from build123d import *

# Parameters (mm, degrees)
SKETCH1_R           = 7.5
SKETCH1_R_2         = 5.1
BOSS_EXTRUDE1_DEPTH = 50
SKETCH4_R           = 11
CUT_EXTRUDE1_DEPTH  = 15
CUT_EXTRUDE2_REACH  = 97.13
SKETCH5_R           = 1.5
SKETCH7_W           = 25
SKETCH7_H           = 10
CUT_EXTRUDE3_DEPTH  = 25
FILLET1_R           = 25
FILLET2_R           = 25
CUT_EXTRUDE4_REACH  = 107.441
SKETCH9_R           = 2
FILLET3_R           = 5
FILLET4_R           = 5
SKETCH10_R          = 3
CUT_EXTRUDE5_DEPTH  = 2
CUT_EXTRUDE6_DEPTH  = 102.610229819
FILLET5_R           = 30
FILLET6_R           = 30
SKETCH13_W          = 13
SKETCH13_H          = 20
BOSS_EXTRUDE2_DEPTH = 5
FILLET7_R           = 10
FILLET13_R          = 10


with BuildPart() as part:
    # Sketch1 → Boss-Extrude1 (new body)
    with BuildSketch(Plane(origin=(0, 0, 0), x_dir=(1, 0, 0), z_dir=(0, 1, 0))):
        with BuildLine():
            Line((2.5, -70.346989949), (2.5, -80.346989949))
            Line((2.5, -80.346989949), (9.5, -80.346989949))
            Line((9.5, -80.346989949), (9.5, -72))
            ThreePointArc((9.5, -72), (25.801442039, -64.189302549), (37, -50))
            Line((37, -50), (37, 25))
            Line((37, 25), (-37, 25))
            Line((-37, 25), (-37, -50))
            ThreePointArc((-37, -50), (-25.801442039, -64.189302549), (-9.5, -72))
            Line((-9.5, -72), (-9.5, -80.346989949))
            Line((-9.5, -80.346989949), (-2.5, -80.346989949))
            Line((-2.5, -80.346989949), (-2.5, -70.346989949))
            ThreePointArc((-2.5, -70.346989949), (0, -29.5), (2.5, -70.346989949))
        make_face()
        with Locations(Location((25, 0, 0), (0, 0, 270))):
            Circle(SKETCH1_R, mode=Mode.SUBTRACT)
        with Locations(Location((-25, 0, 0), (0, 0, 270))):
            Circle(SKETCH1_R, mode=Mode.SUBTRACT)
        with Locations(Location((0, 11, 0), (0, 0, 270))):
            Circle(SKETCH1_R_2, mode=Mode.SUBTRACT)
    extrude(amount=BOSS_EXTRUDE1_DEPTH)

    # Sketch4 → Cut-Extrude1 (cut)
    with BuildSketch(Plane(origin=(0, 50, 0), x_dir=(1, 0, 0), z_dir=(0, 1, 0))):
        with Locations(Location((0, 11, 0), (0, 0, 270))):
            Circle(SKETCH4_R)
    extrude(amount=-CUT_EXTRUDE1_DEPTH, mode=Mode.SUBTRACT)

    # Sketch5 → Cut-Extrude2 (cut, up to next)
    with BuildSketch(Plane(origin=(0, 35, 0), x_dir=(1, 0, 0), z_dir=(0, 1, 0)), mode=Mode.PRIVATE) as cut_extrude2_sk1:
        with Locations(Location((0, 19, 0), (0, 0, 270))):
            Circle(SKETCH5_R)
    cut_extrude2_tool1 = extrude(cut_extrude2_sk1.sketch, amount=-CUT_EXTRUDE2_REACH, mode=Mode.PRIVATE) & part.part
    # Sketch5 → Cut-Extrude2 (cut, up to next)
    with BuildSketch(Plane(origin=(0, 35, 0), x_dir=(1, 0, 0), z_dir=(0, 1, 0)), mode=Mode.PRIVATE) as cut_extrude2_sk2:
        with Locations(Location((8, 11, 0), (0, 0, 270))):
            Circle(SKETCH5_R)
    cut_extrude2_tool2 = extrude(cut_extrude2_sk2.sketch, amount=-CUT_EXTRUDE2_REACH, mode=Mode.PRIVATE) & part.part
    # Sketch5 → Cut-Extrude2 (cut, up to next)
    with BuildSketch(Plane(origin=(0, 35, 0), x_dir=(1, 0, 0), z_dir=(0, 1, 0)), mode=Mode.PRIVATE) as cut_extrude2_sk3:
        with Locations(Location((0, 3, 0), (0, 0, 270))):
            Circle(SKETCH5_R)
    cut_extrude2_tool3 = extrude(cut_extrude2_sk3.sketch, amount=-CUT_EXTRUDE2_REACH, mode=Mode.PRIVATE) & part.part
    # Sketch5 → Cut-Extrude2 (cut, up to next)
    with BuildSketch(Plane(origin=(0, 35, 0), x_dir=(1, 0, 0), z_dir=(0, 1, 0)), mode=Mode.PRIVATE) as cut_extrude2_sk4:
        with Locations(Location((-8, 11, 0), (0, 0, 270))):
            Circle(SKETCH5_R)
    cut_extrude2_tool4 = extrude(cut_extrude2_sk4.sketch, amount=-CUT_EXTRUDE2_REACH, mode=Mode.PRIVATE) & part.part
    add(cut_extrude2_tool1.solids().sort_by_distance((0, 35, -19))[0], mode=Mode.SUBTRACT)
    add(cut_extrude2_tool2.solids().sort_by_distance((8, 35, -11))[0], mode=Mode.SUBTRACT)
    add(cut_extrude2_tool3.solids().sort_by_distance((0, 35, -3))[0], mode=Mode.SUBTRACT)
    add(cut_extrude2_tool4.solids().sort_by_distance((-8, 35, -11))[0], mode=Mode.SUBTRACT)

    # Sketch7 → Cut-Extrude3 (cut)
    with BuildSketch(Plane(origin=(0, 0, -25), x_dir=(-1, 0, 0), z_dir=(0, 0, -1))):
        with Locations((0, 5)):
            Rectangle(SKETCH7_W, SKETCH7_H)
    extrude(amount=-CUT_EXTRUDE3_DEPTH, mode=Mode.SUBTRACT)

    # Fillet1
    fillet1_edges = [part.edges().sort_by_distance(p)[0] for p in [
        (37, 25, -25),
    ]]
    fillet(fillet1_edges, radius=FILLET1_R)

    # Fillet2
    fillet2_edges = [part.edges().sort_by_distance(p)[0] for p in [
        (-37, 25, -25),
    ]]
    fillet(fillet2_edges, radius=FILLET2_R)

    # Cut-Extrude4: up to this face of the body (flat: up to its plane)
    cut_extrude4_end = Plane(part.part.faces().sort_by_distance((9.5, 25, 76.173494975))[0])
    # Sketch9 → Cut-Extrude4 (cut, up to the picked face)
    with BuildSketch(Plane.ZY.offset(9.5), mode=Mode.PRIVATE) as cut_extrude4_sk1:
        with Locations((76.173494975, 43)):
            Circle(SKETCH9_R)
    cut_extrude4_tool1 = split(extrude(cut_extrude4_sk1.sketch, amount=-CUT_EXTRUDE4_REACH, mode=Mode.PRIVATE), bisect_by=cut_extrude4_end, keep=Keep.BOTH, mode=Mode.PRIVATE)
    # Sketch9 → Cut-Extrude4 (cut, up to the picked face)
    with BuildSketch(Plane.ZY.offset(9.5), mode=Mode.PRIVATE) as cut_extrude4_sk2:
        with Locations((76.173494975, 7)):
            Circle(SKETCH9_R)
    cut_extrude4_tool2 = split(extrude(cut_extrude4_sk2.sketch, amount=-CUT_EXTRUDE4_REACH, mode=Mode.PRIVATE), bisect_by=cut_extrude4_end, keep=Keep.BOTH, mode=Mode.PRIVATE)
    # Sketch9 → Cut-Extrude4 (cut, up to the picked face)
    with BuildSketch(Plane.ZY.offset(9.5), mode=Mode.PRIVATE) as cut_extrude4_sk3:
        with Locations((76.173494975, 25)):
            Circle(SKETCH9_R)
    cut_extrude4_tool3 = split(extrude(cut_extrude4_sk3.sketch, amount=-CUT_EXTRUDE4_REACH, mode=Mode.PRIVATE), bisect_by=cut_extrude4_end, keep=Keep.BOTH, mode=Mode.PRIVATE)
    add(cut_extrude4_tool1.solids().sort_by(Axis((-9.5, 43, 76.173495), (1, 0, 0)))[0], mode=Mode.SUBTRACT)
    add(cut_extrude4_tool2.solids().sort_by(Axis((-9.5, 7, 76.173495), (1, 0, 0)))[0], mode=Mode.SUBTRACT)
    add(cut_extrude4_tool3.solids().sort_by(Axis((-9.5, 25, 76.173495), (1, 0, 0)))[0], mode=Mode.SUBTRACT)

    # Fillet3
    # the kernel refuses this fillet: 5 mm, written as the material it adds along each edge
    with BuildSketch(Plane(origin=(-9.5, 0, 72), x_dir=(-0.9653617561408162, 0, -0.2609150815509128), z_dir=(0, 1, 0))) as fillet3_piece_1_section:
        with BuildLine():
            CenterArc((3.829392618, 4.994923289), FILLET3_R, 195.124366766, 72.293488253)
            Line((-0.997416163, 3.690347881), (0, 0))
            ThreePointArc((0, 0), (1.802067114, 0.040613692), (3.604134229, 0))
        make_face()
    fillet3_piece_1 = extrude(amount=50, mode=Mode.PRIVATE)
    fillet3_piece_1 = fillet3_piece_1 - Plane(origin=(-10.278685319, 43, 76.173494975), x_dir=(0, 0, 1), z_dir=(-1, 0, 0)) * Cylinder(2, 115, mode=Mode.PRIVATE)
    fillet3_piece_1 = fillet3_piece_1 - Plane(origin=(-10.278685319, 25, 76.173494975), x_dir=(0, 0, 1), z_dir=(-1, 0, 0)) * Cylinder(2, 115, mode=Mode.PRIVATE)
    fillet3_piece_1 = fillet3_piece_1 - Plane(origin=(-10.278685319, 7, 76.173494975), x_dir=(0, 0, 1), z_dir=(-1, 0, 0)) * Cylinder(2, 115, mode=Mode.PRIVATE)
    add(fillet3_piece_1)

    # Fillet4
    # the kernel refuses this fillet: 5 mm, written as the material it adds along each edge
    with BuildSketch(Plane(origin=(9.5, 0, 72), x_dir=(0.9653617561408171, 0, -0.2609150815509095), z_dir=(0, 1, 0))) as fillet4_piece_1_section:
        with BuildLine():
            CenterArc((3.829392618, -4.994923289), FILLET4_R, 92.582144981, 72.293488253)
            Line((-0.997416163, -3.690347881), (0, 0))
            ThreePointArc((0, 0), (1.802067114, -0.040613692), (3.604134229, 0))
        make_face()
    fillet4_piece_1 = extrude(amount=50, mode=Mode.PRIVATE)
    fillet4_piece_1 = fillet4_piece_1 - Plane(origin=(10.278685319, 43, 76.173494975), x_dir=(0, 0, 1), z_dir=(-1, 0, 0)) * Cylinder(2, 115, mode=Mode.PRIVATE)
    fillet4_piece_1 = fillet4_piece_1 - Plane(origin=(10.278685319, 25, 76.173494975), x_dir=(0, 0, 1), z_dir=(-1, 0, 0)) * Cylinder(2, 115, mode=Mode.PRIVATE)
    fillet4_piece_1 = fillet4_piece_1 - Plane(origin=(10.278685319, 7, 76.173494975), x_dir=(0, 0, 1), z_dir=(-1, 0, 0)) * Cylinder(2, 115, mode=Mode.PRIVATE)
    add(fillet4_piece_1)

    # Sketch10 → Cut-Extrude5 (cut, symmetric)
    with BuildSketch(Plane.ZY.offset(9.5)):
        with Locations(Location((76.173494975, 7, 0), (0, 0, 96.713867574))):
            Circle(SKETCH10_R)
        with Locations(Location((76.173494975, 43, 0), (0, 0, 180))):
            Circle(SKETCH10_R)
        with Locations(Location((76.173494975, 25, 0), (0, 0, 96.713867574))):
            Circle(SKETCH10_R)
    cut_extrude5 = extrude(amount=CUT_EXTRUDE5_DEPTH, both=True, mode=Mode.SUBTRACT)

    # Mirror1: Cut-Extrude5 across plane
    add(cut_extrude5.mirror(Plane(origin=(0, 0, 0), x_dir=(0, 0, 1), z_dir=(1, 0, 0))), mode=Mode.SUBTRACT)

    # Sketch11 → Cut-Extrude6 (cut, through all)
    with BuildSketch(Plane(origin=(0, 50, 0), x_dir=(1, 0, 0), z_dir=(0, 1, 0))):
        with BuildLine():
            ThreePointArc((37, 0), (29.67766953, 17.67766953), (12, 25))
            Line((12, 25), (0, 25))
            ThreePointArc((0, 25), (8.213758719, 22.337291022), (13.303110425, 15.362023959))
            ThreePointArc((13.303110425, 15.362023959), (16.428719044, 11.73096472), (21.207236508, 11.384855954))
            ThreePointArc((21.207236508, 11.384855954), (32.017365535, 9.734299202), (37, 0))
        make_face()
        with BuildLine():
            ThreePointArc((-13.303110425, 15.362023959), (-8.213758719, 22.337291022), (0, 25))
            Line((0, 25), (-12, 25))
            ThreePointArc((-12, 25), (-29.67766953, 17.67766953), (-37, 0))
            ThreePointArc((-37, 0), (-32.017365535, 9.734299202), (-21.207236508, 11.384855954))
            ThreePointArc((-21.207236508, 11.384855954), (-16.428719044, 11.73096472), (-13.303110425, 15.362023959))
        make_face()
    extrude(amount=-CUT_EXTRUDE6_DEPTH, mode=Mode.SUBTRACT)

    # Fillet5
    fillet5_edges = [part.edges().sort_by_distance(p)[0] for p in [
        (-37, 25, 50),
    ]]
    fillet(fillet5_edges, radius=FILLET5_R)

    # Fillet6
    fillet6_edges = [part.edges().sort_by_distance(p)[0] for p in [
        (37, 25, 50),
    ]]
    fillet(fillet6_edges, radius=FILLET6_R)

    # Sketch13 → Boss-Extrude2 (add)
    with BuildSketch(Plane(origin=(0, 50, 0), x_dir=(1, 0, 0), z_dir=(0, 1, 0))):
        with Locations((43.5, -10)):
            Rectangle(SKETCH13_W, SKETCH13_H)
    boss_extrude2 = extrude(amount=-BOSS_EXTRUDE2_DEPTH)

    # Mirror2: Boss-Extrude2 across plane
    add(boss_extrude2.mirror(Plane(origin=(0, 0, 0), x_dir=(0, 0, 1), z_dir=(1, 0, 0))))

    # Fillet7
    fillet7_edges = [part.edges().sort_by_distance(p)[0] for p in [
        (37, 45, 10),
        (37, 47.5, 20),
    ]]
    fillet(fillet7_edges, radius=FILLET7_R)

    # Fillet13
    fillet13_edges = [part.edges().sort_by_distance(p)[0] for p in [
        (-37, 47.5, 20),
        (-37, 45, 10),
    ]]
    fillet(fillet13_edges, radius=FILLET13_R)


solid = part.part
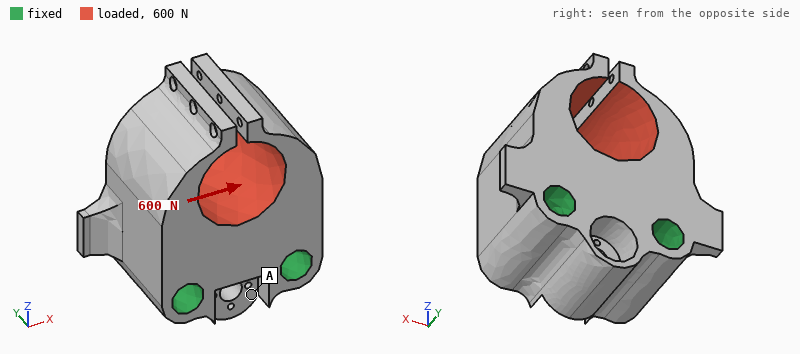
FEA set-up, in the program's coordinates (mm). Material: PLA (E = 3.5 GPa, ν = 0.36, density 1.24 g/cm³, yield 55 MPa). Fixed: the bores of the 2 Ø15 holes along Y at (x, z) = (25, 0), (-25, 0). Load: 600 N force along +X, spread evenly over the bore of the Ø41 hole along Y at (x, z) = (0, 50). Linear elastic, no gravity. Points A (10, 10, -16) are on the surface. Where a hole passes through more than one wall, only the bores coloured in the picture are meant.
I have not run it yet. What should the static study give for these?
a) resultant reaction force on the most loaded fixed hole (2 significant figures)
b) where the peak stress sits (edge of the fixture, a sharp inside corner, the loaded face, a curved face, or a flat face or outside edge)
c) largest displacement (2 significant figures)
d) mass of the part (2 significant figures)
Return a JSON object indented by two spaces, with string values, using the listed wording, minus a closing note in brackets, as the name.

{
  "resultant reaction force on the most loaded fixed hole": "540 N",
  "where the peak stress sits": "the loaded face",
  "largest displacement": "85 µm",
  "mass of the part": "260 g"
}
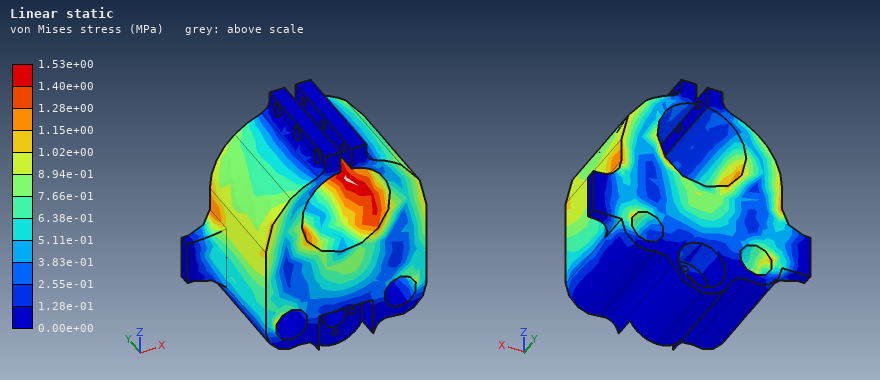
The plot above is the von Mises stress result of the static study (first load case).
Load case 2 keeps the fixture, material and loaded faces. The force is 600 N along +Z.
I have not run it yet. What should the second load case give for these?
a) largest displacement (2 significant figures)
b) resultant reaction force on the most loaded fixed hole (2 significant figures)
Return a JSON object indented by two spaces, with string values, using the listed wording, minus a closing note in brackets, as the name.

{
  "largest displacement": "0.10 mm",
  "resultant reaction force on the most loaded fixed hole": "330 N"
}
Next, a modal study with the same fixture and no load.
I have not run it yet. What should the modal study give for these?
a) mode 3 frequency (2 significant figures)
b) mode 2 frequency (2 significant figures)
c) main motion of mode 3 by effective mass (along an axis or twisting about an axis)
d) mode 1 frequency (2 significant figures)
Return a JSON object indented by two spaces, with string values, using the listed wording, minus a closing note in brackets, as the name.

{
  "mode 3 frequency": "2400 Hz",
  "mode 2 frequency": "1600 Hz",
  "main motion of mode 3 by effective mass": "along Y",
  "mode 1 frequency": "1600 Hz"
}
